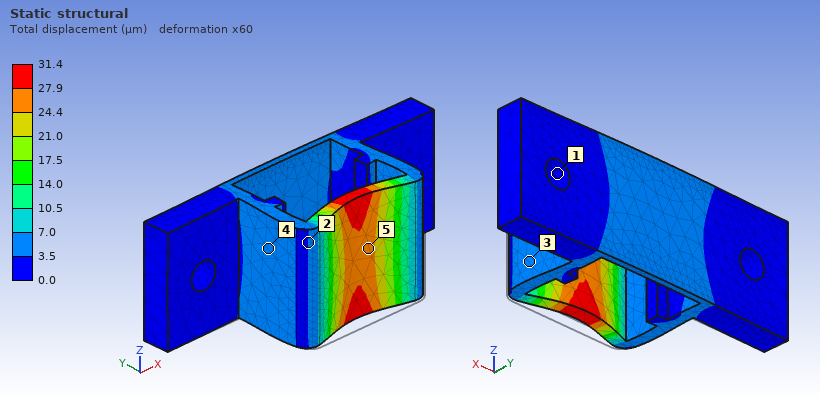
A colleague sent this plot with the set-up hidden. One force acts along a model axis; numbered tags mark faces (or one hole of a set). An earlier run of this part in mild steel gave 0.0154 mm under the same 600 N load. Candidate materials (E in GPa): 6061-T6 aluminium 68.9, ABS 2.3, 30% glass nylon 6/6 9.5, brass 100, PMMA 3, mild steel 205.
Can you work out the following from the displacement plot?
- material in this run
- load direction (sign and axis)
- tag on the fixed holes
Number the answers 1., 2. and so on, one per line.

1. brass
2. +Y
3. 1
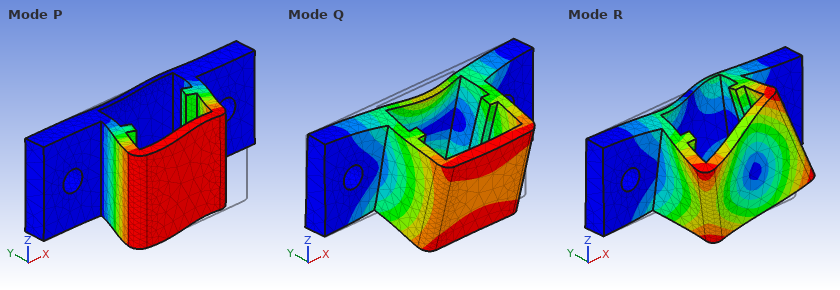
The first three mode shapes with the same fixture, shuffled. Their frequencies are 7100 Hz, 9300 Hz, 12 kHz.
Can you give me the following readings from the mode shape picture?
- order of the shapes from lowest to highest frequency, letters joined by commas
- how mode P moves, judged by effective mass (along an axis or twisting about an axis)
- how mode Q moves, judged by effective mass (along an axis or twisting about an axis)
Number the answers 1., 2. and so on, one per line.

1. P, Q, R
2. along X
3. along Z
